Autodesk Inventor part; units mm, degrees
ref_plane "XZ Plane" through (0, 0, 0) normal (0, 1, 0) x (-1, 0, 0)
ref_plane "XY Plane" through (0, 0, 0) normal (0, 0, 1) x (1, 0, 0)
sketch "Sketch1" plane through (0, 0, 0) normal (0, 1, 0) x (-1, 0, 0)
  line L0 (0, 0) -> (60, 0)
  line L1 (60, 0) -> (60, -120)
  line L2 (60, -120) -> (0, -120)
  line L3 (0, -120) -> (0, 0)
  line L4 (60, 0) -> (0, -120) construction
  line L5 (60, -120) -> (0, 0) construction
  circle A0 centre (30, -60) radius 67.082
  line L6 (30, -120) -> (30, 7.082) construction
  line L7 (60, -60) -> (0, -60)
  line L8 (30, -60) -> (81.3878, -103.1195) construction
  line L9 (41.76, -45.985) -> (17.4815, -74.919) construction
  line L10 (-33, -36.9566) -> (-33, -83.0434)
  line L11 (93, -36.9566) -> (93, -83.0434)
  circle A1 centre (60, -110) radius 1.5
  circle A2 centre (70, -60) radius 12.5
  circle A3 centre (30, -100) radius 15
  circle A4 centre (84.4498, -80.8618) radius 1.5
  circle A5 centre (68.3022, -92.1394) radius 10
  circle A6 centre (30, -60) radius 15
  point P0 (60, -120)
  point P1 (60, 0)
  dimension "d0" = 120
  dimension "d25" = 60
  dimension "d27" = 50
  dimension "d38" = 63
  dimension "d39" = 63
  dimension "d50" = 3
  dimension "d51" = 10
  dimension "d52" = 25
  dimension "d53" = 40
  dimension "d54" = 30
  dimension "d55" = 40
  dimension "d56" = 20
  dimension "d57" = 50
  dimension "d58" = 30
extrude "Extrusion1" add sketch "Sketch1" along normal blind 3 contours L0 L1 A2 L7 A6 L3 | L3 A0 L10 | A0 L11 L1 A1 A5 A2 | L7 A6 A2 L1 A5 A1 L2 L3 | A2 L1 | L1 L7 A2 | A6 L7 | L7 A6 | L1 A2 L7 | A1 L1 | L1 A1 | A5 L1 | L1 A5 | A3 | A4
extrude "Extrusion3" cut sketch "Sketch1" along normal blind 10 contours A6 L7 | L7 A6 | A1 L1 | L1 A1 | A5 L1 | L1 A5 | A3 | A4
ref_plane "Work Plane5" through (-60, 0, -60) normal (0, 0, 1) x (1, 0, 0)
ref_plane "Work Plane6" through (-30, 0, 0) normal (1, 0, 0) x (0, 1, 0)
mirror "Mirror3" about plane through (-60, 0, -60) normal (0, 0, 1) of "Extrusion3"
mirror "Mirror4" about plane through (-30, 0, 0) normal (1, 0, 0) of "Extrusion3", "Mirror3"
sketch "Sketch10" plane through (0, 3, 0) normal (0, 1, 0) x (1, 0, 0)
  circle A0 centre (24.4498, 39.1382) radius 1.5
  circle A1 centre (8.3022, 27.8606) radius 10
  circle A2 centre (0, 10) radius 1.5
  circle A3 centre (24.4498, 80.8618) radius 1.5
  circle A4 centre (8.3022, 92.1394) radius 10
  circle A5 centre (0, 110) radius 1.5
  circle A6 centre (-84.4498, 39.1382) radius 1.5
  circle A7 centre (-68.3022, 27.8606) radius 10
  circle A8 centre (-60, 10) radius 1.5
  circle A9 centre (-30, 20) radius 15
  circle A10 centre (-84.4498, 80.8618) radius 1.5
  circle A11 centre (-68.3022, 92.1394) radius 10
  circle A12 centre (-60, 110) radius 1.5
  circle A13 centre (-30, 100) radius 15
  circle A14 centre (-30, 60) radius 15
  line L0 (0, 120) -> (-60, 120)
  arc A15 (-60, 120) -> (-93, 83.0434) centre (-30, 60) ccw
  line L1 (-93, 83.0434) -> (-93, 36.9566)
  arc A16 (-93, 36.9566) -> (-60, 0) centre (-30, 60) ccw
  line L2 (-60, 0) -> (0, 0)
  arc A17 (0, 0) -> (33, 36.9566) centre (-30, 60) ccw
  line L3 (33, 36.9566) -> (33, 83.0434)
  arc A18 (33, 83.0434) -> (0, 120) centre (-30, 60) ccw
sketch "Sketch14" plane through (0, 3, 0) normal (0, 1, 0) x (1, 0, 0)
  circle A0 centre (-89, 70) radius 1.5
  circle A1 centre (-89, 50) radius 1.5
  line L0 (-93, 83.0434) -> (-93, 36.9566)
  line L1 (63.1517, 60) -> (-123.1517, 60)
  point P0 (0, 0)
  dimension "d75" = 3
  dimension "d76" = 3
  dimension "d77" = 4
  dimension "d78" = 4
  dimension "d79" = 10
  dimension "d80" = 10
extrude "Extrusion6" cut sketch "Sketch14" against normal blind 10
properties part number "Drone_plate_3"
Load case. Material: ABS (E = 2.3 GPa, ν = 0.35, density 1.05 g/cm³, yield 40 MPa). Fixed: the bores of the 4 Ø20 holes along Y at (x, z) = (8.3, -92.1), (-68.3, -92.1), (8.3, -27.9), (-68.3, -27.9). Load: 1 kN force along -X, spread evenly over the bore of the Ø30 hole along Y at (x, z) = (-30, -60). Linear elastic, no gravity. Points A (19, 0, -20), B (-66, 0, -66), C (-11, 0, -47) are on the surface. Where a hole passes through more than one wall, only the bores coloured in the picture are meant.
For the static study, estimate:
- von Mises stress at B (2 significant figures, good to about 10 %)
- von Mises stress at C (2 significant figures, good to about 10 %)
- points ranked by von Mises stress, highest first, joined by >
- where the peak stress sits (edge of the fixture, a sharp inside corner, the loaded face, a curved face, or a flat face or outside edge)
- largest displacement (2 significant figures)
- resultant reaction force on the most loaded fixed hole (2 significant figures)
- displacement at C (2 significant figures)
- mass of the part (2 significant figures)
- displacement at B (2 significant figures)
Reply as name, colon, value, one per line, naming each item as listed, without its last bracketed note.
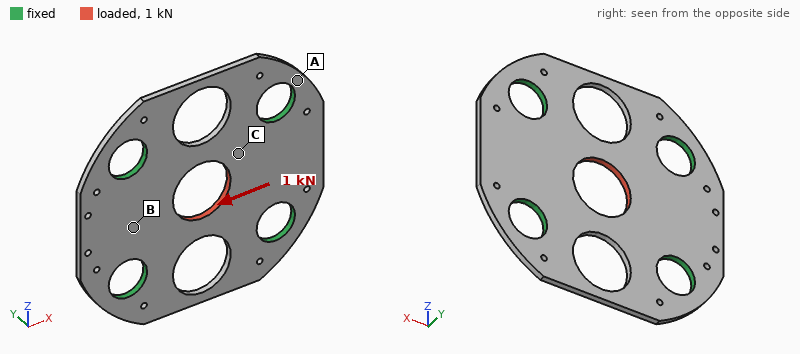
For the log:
von Mises stress at B: 1.6 MPa
von Mises stress at C: 3.0 MPa
points ranked by von Mises stress, highest first, joined by >: C > B > A
where the peak stress sits: a sharp inside corner
largest displacement: 53 µm
resultant reaction force on the most loaded fixed hole: 270 N
displacement at C: 34 µm
mass of the part: 31 g
displacement at B: 30 µm
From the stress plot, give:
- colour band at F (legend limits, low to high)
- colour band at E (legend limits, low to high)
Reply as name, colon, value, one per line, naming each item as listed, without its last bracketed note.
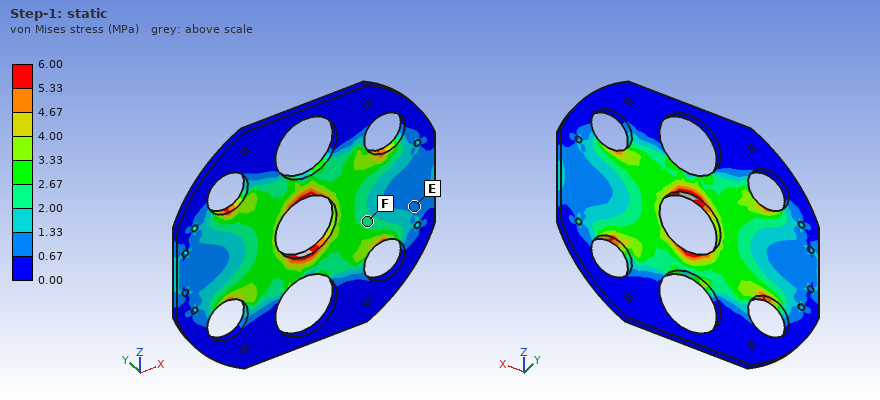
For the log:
colour band at F: 2.00 to 2.67 MPa
colour band at E: 0.67 to 1.33 MPa
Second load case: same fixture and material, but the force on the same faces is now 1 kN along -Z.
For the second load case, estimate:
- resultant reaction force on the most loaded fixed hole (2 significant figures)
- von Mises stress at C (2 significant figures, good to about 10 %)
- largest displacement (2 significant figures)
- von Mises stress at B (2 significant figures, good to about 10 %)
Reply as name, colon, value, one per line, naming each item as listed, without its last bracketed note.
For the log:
resultant reaction force on the most loaded fixed hole: 290 N
von Mises stress at C: 3.8 MPa
largest displacement: 91 µm
von Mises stress at B: 1.4 MPa
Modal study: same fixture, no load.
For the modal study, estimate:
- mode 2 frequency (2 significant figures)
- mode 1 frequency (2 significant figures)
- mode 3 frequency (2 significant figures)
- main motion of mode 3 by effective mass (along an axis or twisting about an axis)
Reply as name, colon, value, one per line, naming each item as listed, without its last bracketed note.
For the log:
mode 2 frequency: 1000 Hz
mode 1 frequency: 1000 Hz
mode 3 frequency: 1200 Hz
main motion of mode 3 by effective mass: along Y
